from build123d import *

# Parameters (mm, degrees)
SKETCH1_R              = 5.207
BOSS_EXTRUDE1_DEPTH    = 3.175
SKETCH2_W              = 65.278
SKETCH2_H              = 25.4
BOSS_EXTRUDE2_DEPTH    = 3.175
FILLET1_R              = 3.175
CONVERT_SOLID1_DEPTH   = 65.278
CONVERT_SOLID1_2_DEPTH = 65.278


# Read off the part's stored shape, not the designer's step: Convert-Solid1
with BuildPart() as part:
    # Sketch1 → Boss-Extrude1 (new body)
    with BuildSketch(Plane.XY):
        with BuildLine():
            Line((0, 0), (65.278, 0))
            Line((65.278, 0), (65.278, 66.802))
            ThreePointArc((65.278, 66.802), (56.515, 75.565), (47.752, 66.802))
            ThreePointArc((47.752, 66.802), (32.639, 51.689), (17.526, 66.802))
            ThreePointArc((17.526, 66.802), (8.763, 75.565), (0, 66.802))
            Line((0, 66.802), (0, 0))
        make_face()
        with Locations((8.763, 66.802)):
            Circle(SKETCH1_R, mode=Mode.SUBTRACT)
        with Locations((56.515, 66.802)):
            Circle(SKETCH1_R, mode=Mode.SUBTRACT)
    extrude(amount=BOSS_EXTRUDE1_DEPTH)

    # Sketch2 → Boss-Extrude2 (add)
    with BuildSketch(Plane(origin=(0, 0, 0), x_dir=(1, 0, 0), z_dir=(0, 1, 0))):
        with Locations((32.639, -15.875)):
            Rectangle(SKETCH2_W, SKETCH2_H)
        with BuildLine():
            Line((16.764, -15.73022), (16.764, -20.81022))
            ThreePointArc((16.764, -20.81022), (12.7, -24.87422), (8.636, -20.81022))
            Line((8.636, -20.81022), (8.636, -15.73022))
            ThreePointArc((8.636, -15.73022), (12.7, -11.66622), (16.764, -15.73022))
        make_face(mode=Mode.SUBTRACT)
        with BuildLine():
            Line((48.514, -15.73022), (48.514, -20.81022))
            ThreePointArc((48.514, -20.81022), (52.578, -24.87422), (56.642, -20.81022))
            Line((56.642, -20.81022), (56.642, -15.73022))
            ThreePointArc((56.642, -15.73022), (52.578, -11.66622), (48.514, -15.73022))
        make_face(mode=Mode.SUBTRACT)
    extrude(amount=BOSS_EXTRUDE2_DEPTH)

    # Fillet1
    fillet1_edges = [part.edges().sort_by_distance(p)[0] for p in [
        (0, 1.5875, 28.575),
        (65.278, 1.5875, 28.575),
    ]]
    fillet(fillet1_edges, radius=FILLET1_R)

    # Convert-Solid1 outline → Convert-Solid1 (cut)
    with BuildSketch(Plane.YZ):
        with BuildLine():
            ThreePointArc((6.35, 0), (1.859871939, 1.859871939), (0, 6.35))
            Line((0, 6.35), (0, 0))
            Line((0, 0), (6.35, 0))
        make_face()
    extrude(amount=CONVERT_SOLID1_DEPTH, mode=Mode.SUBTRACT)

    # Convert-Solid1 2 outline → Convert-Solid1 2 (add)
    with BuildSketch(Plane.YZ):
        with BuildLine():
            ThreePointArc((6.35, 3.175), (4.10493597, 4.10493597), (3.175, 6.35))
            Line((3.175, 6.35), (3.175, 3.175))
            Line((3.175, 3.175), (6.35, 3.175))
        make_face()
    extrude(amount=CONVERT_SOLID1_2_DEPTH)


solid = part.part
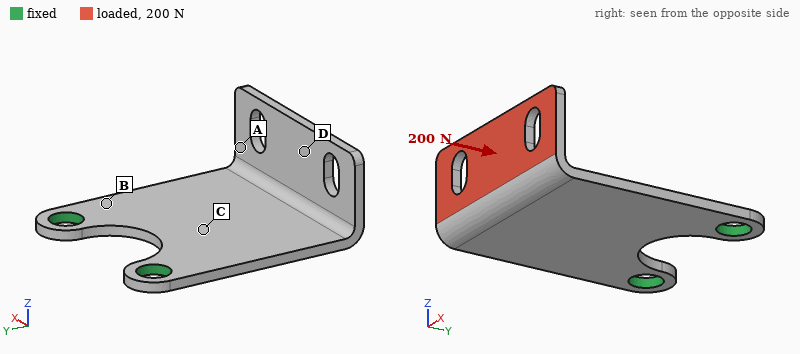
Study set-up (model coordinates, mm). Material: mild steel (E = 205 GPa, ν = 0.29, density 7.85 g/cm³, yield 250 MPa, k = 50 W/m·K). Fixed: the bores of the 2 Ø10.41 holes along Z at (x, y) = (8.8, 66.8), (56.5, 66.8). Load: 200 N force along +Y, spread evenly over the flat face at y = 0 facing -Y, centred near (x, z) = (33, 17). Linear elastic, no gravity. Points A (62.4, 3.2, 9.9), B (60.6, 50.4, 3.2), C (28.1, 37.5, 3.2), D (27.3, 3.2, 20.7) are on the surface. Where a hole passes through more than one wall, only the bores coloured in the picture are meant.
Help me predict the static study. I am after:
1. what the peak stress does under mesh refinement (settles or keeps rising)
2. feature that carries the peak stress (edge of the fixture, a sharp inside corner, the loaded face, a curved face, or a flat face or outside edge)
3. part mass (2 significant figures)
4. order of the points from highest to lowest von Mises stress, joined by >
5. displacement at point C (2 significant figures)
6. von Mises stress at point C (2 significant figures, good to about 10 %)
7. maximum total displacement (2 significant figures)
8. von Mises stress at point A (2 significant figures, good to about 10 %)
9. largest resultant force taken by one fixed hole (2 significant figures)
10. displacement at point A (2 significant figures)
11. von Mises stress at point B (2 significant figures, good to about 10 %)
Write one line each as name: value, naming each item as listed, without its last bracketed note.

what the peak stress does under mesh refinement: keeps rising
feature that carries the peak stress: edge of the fixture
part mass: 130 g
order of the points from highest to lowest von Mises stress, joined by >: B > C > A > D
displacement at point C: 0.044 mm
von Mises stress at point C: 25 MPa
maximum total displacement: 0.27 mm
von Mises stress at point A: 13 MPa
largest resultant force taken by one fixed hole: 100 N
displacement at point A: 0.20 mm
von Mises stress at point B: 39 MPa
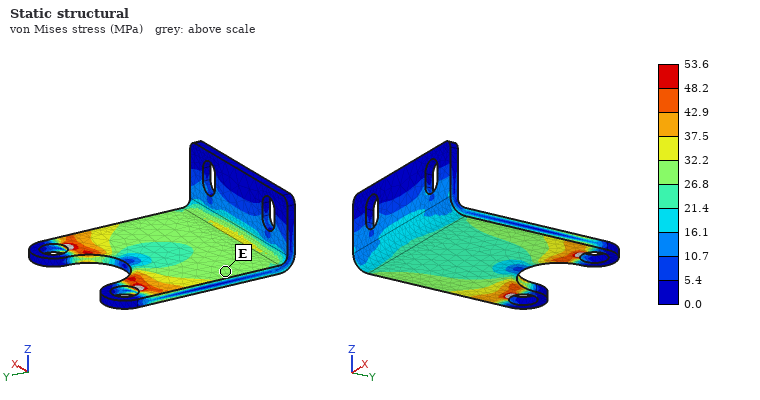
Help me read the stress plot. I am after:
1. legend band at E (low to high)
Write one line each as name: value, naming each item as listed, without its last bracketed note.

legend band at E: 26.8 to 32.2 MPa
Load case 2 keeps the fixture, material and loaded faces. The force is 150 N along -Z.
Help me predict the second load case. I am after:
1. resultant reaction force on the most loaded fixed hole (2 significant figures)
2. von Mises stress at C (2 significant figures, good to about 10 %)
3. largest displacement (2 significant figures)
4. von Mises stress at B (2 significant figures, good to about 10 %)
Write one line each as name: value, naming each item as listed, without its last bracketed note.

resultant reaction force on the most loaded fixed hole: 75 N
von Mises stress at C: 43 MPa
largest displacement: 0.53 mm
von Mises stress at B: 93 MPa
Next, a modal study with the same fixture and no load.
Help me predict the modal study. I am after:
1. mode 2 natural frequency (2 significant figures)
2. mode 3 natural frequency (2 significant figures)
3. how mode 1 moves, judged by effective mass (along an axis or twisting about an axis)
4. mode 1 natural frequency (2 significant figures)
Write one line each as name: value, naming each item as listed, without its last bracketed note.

mode 2 natural frequency: 1000 Hz
mode 3 natural frequency: 1900 Hz
how mode 1 moves, judged by effective mass: along Z
mode 1 natural frequency: 370 Hz
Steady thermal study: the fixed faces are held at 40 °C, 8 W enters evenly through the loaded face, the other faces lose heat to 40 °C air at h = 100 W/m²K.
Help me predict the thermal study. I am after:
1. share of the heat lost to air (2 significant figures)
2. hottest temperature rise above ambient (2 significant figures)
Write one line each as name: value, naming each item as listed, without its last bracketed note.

share of the heat lost to air: 91 %
hottest temperature rise above ambient: 19 K
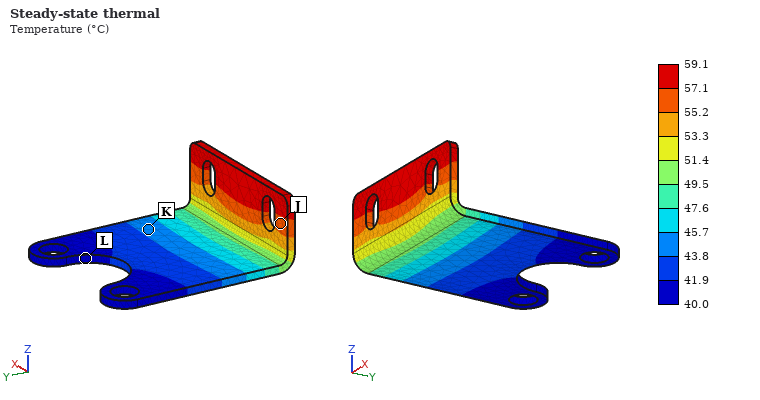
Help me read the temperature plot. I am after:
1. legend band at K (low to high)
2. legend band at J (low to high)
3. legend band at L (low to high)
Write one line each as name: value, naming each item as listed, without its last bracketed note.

legend band at K: 43.8 to 45.7 °C
legend band at J: 55.2 to 57.1 °C
legend band at L: 40.0 to 41.9 °C
